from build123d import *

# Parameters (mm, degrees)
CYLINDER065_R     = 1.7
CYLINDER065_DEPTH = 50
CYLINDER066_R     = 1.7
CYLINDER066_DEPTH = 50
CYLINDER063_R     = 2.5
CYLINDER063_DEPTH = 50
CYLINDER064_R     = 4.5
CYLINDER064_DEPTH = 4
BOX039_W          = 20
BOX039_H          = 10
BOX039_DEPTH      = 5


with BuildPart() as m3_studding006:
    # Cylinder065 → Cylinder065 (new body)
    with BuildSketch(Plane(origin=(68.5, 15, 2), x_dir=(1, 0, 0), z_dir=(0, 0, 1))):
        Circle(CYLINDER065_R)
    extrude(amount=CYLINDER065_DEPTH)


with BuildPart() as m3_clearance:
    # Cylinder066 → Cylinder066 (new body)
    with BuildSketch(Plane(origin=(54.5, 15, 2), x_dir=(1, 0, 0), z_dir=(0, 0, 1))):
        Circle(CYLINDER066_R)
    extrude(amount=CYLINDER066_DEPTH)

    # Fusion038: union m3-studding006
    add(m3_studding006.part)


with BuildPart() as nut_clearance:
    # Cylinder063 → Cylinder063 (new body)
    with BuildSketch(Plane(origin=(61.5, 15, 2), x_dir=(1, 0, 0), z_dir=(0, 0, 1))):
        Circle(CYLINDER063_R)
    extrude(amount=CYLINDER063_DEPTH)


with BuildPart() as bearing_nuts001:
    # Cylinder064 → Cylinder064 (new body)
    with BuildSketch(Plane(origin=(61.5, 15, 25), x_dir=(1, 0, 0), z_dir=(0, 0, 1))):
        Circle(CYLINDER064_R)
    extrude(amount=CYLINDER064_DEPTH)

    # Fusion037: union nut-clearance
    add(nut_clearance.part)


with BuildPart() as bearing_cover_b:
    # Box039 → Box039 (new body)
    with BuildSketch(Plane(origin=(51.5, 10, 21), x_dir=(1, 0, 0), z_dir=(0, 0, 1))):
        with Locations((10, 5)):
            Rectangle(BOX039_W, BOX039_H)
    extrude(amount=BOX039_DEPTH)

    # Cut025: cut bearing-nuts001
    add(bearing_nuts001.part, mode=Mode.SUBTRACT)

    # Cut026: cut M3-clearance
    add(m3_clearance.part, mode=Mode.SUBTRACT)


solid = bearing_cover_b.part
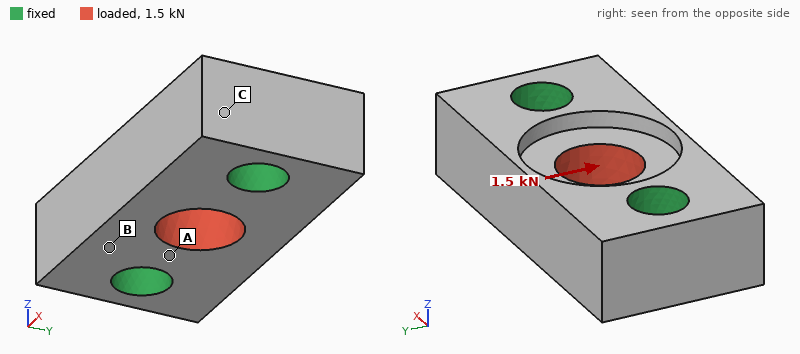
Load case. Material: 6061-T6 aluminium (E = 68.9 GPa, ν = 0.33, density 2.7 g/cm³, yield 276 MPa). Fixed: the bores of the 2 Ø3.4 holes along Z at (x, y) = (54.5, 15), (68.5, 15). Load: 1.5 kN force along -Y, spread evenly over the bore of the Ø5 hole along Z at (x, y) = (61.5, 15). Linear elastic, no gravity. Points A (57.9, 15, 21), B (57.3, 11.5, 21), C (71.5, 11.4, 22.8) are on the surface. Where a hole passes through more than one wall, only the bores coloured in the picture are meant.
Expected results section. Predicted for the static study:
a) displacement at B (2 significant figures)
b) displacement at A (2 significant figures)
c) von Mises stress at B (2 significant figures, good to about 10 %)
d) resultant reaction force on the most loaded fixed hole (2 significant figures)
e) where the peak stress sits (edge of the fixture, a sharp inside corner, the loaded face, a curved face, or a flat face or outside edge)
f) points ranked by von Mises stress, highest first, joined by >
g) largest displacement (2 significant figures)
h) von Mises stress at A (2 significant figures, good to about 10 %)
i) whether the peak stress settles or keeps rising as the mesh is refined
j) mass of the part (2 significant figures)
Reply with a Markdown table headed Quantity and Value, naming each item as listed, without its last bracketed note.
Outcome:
| Quantity | Value |
|---|---|
| displacement at B | 2.3 µm |
| displacement at A | 2.7 µm |
| von Mises stress at B | 27 MPa |
| resultant reaction force on the most loaded fixed hole | 750 N |
| where the peak stress sits | edge of the fixture |
| points ranked by von Mises stress, highest first, joined by > | A > B > C |
| largest displacement | 6.0 µm |
| von Mises stress at A | 49 MPa |
| whether the peak stress settles or keeps rising as the mesh is refined | keeps rising |
| mass of the part | 2.1 g |
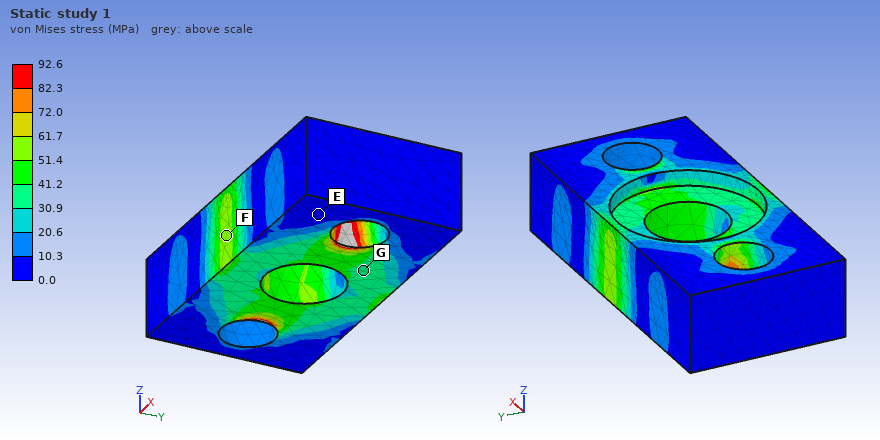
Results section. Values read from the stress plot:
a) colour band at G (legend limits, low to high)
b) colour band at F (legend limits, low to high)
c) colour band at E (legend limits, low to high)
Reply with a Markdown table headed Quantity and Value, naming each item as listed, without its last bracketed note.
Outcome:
| Quantity | Value |
|---|---|
| colour band at G | 30.9 to 41.2 MPa |
| colour band at F | 51.4 to 61.7 MPa |
| colour band at E | 0.0 to 10.3 MPa |
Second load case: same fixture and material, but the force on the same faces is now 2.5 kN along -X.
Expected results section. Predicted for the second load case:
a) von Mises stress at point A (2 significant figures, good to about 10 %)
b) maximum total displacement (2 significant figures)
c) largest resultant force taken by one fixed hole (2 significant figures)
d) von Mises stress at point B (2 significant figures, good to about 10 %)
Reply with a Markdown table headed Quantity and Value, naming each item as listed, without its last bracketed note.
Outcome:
| Quantity | Value |
|---|---|
| von Mises stress at point A | 53 MPa |
| maximum total displacement | 3.9 µm |
| largest resultant force taken by one fixed hole | 1.3 kN |
| von Mises stress at point B | 20 MPa |
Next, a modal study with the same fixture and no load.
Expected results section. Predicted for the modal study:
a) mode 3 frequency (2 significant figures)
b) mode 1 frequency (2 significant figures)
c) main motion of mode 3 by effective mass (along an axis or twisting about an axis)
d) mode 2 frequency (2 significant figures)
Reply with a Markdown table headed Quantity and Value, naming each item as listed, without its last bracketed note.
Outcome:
| Quantity | Value |
|---|---|
| mode 3 frequency | 110 kHz |
| mode 1 frequency | 90 kHz |
| main motion of mode 3 by effective mass | along Y |
| mode 2 frequency | 92 kHz |
